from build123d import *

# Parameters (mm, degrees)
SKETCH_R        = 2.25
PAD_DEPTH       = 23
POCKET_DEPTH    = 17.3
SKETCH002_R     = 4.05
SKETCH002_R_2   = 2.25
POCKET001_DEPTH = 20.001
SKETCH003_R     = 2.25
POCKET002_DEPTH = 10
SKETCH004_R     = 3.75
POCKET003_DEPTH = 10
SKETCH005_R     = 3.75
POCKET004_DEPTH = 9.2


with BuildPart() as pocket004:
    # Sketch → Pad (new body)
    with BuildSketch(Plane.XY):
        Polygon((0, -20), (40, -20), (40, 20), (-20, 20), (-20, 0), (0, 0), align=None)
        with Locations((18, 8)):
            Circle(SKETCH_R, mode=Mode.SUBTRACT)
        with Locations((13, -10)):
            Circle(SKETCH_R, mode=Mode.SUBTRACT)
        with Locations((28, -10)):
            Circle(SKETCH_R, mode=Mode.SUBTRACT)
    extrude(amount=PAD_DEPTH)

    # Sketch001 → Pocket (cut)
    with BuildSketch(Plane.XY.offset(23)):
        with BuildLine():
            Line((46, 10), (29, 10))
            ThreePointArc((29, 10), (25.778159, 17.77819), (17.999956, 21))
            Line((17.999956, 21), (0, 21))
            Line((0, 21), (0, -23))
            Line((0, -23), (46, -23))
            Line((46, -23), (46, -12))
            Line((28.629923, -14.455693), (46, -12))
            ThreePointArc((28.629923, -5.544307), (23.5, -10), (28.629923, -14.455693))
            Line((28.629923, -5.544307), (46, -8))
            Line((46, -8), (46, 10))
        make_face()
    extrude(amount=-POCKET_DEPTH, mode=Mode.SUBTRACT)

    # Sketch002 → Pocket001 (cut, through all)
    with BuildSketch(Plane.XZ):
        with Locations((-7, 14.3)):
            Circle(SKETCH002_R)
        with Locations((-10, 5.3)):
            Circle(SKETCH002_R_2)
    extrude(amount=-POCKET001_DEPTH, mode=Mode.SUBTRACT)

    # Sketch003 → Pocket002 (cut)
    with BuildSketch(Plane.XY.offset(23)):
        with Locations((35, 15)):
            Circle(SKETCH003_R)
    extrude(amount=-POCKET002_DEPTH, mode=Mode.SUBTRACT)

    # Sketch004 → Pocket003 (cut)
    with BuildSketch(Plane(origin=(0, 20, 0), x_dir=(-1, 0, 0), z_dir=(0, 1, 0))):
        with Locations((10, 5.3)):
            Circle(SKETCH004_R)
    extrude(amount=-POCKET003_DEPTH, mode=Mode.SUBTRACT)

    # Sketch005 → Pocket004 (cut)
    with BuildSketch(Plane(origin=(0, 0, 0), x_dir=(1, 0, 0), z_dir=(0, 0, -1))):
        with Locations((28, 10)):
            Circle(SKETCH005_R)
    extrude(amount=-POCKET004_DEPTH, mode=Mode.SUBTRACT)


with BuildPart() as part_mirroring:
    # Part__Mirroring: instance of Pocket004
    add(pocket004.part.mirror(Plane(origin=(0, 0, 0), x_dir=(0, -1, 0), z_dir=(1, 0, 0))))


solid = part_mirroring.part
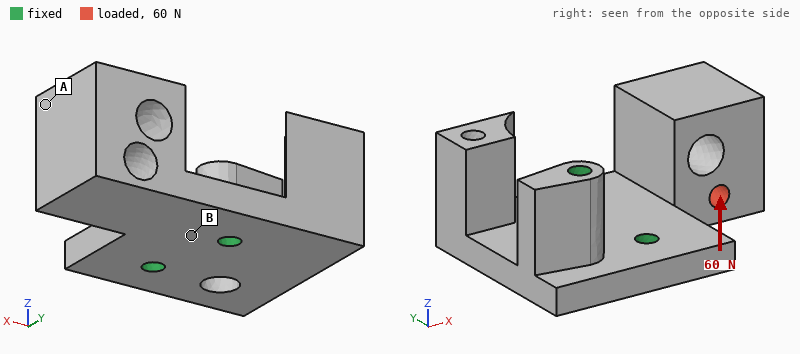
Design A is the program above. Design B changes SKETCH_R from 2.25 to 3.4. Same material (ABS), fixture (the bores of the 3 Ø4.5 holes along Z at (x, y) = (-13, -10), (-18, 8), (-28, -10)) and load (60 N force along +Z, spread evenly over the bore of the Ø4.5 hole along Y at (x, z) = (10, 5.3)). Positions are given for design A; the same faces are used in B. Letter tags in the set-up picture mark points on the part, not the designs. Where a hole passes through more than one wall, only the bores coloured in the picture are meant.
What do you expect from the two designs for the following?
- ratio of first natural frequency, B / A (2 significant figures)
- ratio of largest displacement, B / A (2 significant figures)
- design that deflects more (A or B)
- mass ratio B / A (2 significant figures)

1.1
0.89
A
0.97
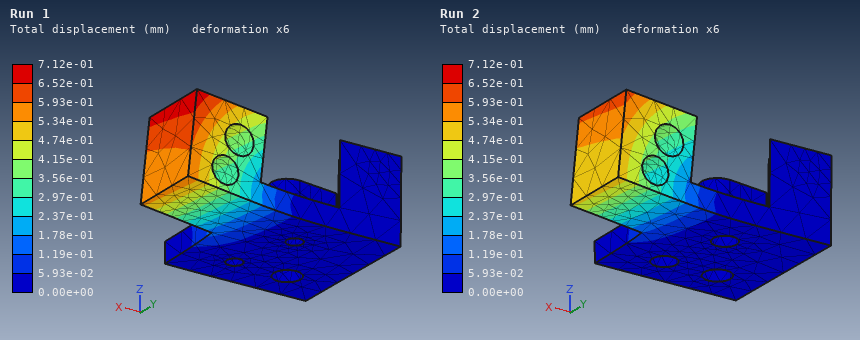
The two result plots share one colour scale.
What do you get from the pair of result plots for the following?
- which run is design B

Run 2
